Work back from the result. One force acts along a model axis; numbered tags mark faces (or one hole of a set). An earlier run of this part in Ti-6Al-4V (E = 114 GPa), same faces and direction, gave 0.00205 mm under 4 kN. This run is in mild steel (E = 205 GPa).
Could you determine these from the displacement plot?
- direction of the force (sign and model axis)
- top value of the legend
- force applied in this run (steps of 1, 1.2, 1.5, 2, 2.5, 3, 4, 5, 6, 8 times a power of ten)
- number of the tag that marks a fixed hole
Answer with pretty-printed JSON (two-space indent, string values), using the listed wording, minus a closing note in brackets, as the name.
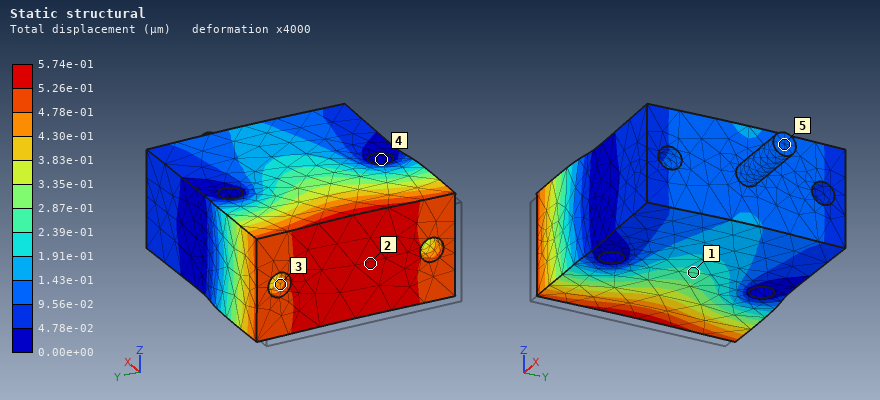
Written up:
{
  "direction of the force": "+X",
  "top value of the legend": "5.74e-01 µm",
  "force applied in this run": "2 kN",
  "number of the tag that marks a fixed hole": "4"
}
